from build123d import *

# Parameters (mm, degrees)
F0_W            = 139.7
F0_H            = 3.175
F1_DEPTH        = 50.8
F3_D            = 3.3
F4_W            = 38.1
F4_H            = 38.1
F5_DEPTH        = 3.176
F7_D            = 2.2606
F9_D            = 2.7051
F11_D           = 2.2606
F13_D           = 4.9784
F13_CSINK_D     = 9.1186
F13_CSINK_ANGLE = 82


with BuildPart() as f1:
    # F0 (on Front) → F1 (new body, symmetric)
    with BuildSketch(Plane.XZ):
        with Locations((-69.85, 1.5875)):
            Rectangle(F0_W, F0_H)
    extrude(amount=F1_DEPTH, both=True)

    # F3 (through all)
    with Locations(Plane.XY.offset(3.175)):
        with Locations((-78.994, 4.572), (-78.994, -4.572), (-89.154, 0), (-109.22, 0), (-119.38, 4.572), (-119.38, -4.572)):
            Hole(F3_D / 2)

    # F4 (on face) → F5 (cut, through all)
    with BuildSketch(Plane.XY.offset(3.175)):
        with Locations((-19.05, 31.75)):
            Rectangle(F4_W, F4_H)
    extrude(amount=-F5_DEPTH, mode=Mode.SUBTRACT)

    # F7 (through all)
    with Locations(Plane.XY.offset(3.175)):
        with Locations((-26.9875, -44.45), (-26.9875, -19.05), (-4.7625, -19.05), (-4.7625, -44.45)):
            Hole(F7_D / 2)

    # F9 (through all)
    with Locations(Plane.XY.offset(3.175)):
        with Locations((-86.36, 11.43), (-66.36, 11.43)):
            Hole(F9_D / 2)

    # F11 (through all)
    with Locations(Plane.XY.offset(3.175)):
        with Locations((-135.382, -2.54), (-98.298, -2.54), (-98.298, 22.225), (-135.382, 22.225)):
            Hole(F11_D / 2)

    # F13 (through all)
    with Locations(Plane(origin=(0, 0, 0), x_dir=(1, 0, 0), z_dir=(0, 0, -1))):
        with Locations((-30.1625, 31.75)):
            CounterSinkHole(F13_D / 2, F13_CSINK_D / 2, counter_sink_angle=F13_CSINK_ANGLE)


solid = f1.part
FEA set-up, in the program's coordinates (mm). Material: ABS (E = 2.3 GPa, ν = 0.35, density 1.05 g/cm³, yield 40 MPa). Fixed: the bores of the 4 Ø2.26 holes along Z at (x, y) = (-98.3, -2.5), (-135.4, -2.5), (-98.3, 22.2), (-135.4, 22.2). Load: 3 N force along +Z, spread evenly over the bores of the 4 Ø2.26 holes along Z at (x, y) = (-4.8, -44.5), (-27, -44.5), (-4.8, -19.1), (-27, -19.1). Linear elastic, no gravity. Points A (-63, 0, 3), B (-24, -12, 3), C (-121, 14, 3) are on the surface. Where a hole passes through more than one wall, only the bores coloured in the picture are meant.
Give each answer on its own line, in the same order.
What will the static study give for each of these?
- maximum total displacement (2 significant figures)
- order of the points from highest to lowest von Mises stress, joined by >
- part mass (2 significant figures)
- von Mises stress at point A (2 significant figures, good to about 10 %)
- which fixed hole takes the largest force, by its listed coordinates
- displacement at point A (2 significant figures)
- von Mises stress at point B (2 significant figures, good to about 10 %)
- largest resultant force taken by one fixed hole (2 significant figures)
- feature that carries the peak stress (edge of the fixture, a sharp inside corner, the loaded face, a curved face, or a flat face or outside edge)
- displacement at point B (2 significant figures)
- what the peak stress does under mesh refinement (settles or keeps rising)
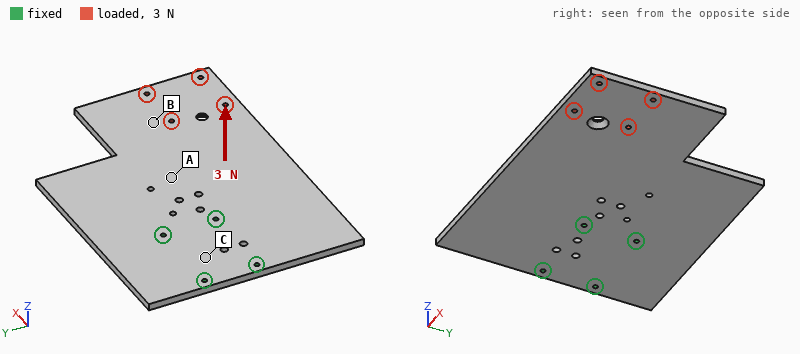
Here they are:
2.0 mm
A > B > C
42 g
0.98 MPa
(-98.3, -2.5)
0.31 mm
0.47 MPa
8.1 N
edge of the fixture
1.1 mm
keeps rising
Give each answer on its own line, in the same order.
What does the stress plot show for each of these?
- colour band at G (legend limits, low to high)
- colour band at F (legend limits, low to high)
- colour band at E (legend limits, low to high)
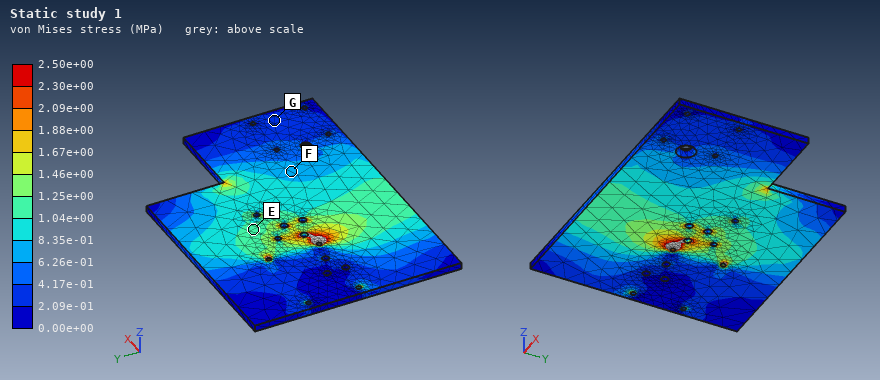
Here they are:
2.09e-01 to 4.17e-01 MPa
6.26e-01 to 8.35e-01 MPa
1.04e+00 to 1.25e+00 MPa
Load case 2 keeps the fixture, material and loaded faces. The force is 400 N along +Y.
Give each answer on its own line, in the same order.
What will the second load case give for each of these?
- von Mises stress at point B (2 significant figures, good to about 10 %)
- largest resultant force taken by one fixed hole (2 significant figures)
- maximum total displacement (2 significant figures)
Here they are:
4.2 MPa
590 N
1.0 mm
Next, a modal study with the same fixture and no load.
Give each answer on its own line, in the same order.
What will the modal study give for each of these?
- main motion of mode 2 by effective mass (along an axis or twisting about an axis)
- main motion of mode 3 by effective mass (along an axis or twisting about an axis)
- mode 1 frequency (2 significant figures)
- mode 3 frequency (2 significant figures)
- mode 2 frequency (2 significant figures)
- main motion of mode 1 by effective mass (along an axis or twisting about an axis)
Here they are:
twisting about X
along Z
81 Hz
320 Hz
200 Hz
along Z
